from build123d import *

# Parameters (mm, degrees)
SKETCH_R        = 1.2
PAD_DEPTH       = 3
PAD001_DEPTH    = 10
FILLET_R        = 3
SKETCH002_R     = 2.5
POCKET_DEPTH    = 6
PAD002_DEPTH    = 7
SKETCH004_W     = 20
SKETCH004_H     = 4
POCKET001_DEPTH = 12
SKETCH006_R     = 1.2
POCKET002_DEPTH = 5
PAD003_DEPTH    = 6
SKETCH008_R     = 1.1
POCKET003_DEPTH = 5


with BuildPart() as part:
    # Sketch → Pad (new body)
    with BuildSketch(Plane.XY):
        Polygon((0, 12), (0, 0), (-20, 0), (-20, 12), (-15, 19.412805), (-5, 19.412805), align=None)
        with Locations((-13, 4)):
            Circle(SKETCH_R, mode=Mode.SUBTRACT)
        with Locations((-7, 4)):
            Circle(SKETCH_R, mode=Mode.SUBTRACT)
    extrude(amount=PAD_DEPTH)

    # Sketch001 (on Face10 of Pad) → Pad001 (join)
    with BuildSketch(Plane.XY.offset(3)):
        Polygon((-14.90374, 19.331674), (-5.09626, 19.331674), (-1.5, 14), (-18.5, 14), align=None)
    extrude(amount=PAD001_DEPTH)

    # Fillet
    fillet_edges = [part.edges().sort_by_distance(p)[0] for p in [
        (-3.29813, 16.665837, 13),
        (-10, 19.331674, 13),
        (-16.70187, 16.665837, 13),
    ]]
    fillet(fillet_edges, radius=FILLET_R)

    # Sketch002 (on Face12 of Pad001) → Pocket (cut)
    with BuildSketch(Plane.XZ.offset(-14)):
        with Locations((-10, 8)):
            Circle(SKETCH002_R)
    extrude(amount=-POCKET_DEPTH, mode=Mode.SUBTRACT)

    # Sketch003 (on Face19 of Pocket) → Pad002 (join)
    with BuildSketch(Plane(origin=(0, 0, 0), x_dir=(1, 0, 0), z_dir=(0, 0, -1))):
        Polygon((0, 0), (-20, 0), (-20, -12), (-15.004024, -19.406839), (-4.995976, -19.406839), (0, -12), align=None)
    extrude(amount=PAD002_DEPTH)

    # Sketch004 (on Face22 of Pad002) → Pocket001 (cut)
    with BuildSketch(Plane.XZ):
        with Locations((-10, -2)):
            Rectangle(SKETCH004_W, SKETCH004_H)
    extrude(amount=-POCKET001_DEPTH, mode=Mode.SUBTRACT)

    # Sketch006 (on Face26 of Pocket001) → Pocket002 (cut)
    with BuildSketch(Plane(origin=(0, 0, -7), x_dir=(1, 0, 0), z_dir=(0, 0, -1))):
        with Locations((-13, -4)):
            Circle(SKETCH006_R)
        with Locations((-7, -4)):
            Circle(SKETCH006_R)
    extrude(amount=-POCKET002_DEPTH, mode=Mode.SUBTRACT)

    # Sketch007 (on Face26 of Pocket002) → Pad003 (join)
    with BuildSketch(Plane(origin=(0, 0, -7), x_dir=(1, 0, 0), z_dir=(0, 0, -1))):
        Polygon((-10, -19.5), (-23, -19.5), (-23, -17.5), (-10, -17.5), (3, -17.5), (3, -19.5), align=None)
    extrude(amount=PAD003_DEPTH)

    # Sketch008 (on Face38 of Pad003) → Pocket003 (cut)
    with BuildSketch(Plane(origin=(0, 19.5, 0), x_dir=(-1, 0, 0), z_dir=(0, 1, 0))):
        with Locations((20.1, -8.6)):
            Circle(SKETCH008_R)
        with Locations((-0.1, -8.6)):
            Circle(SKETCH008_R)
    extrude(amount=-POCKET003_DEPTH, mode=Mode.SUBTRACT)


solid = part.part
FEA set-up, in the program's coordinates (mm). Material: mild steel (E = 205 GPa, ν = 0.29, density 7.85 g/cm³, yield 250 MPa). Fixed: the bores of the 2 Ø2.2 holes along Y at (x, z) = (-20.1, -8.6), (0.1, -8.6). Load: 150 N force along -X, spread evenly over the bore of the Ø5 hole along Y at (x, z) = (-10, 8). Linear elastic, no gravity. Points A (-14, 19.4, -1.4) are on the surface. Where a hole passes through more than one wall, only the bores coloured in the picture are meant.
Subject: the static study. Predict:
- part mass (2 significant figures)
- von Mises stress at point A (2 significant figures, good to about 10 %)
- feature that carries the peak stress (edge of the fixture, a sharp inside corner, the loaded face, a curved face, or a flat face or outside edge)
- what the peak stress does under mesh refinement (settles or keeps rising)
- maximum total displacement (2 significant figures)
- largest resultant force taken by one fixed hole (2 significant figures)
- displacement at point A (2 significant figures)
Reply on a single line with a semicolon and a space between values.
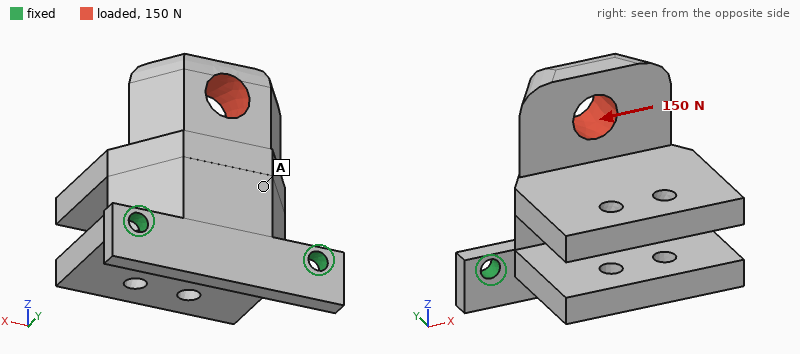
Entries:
26 g; 12 MPa; a sharp inside corner; keeps rising; 8.9 µm; 170 N; 3.2 µm
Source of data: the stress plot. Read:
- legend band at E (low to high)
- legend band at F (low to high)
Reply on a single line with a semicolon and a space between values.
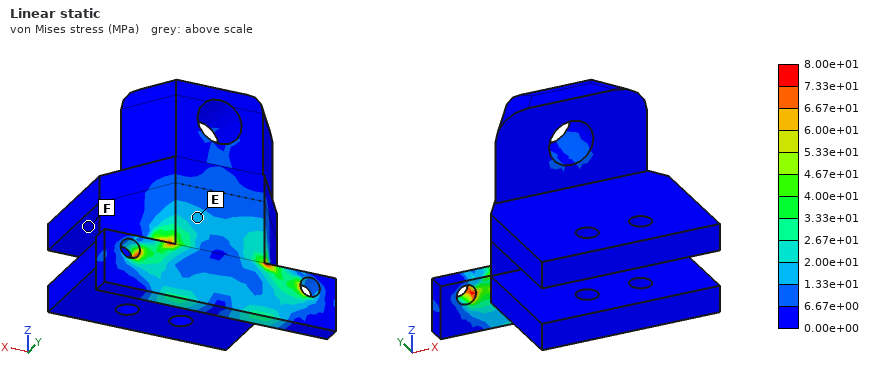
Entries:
1.33e+01 to 2.00e+01 MPa; 0.00e+00 to 6.67e+00 MPa
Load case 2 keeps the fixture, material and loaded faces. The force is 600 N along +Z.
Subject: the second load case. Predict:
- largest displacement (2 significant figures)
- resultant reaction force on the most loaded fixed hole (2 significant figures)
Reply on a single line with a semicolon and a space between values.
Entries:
96 µm; 300 N
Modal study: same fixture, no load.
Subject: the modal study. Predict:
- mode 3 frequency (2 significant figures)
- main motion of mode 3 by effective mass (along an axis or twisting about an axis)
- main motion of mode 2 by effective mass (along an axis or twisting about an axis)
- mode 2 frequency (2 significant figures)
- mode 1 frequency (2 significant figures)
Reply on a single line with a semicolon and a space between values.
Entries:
7900 Hz; along X; along X; 4800 Hz; 1200 Hz
